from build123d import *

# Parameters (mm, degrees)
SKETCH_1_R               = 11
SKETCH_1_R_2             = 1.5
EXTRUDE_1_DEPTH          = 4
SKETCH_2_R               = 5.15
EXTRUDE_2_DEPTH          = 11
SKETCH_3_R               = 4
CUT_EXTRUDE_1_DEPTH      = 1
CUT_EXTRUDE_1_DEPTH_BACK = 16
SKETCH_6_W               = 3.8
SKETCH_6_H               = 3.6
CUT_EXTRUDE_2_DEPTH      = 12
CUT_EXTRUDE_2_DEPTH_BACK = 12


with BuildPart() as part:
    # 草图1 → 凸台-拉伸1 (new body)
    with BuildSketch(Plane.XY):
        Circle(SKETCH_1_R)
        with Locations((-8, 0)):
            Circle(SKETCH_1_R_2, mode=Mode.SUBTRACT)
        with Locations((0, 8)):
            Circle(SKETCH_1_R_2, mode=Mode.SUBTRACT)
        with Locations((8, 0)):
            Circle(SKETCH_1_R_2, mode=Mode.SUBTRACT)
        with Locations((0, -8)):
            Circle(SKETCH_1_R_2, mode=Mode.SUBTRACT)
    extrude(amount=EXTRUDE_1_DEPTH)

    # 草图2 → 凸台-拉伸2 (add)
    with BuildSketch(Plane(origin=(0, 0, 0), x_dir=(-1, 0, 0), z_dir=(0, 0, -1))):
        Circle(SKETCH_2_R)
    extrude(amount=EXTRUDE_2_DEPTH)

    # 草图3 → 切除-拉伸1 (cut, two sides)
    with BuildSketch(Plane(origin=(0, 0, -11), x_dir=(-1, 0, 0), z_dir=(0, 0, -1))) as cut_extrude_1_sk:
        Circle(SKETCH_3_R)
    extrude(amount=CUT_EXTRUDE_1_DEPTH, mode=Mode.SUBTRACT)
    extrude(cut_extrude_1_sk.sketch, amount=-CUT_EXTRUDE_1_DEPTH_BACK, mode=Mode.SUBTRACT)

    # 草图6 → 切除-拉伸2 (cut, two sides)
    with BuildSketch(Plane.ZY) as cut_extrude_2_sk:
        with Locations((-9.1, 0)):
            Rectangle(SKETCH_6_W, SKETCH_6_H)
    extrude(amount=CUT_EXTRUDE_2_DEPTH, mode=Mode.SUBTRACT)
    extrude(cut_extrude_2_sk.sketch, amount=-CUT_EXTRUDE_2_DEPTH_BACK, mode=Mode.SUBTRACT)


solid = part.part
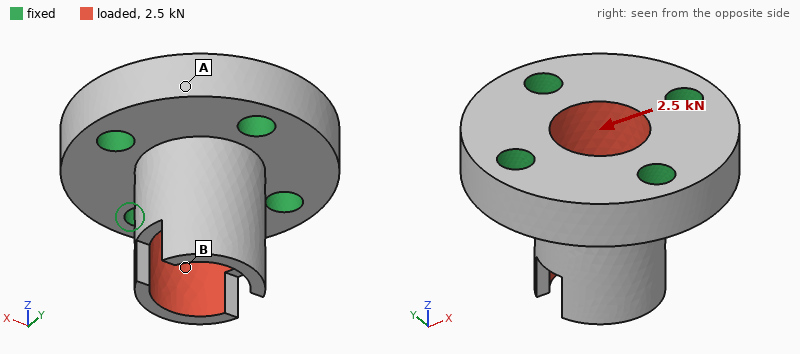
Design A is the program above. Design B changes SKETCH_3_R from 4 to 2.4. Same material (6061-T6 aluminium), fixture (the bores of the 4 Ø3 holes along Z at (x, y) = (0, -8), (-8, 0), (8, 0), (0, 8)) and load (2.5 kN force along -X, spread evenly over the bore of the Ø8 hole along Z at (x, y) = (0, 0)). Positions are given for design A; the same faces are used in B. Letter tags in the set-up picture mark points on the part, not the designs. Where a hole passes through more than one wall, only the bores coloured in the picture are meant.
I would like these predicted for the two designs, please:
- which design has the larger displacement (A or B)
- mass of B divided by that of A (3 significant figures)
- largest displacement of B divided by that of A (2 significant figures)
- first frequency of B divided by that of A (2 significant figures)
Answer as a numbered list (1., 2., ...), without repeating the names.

1. A
2. 1.28
3. 0.39
4. 1.1
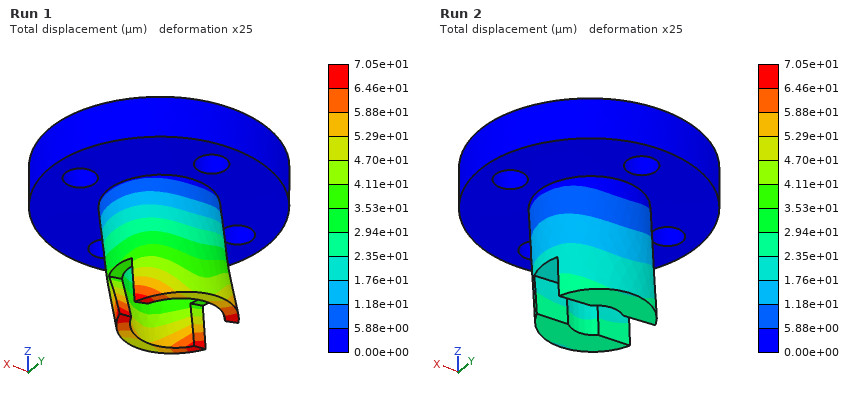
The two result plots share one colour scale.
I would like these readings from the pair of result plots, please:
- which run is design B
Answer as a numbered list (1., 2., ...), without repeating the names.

1. Run 2
